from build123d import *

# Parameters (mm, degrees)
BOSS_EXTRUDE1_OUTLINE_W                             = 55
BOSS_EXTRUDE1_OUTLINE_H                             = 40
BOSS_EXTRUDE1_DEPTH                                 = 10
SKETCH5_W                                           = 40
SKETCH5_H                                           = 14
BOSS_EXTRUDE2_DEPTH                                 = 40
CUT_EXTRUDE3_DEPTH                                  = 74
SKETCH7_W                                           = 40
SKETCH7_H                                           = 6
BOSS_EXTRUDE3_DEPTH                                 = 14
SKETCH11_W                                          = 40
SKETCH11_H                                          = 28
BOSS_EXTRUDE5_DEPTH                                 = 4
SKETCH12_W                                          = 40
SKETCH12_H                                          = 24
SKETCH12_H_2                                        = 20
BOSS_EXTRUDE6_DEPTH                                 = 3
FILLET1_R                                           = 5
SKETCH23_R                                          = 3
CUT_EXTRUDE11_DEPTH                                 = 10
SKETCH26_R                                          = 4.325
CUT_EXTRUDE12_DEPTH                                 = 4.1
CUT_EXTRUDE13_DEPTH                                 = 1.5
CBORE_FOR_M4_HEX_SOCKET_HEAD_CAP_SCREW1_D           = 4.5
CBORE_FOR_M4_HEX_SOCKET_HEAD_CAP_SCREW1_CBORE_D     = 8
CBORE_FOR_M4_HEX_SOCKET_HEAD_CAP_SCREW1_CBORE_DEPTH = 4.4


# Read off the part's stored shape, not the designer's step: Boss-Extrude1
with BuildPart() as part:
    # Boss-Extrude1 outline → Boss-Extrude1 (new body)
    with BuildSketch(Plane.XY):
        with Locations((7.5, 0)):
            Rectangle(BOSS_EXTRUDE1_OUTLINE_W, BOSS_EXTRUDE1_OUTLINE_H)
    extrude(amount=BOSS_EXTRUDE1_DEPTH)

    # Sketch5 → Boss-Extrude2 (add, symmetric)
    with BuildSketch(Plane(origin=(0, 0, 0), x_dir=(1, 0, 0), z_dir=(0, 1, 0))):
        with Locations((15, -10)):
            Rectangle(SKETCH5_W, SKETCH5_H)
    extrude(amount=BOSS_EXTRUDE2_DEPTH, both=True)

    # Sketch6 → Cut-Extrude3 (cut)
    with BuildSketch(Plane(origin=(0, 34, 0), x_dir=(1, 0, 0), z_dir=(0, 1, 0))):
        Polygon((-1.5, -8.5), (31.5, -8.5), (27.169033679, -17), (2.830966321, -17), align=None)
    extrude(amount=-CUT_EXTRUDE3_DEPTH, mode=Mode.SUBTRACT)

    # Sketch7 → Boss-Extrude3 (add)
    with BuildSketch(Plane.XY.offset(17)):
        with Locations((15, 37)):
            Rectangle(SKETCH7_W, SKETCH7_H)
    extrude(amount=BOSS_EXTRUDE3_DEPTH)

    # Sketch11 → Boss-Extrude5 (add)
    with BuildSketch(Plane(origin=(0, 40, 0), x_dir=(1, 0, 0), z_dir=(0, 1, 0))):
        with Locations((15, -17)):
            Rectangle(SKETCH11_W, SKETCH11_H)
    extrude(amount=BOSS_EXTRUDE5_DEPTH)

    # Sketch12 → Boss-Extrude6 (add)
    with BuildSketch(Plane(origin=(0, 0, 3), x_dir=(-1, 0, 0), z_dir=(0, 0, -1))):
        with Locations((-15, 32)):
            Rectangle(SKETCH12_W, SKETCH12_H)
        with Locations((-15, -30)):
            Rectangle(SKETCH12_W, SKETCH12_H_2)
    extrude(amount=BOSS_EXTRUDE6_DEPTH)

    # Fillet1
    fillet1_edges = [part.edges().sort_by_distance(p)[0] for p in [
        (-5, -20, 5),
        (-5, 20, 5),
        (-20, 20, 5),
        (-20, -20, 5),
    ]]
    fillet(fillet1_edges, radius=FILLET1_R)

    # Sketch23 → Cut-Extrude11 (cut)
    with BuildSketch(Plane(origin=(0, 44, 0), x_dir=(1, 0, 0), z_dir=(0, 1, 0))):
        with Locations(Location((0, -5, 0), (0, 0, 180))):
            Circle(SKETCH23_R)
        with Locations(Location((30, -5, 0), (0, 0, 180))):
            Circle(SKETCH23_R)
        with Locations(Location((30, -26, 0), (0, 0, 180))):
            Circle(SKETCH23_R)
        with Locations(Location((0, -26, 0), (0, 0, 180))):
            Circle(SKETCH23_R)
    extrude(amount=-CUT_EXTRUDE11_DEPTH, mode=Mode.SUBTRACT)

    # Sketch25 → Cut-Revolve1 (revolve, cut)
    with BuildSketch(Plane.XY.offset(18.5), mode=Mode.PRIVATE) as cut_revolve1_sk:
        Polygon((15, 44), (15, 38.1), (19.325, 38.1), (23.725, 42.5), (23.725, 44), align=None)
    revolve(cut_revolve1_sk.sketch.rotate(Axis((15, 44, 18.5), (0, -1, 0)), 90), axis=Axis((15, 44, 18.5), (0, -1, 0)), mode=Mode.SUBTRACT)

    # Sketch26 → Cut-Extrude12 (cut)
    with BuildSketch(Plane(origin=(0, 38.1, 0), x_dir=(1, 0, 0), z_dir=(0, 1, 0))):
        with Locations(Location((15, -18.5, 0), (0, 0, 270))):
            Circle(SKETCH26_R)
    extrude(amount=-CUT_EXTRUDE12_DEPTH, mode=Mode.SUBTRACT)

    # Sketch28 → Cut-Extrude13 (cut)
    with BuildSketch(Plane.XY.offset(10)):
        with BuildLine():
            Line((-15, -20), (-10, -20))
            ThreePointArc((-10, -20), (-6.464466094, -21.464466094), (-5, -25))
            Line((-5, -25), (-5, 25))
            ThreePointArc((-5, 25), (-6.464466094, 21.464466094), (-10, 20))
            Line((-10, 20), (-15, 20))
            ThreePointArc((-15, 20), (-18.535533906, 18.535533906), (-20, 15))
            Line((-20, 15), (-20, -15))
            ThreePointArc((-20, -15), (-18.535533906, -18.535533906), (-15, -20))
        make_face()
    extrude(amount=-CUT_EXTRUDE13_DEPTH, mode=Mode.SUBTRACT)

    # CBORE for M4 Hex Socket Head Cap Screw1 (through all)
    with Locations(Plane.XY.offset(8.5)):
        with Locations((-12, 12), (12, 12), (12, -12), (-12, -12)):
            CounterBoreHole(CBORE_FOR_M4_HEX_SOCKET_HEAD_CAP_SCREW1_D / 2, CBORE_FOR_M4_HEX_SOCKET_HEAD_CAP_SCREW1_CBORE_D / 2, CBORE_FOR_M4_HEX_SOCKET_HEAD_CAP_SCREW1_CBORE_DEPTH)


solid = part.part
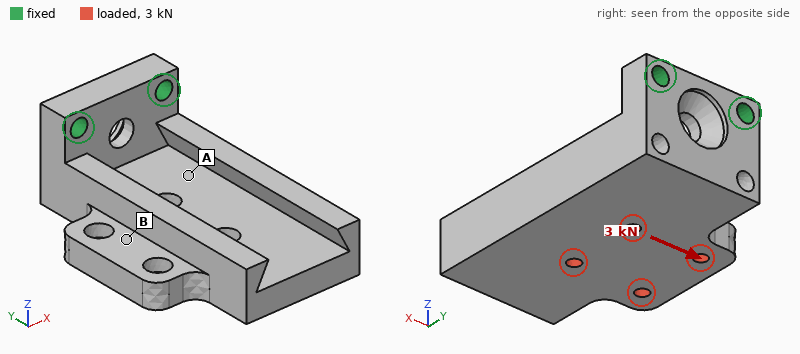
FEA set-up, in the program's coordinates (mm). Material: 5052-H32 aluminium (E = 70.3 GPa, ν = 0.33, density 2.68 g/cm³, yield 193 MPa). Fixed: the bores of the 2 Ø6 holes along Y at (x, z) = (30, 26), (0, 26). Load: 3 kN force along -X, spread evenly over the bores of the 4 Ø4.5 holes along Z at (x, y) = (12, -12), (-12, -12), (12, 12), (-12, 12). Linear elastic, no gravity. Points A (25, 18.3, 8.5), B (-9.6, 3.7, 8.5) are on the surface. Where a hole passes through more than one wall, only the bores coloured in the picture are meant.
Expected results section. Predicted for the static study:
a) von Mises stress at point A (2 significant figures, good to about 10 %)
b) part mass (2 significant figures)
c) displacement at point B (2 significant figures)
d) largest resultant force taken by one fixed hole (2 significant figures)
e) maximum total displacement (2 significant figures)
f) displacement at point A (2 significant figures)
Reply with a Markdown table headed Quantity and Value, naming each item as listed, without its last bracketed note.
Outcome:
| Quantity | Value |
|---|---|
| von Mises stress at point A | 35 MPa |
| part mass | 120 g |
| displacement at point B | 0.14 mm |
| largest resultant force taken by one fixed hole | 4.3 kN |
| maximum total displacement | 0.28 mm |
| displacement at point A | 0.079 mm |
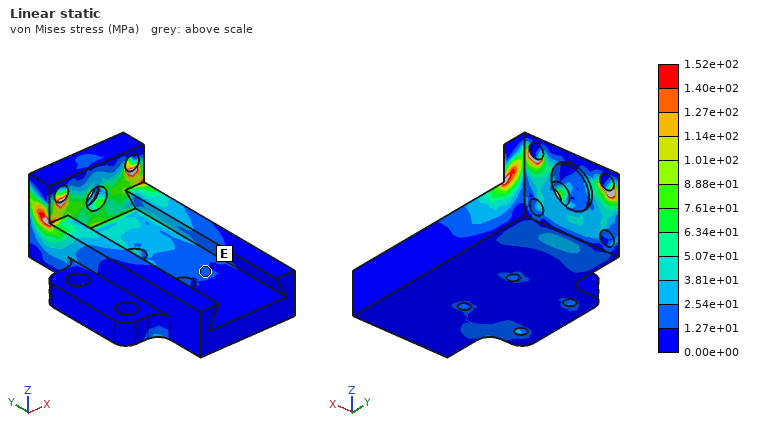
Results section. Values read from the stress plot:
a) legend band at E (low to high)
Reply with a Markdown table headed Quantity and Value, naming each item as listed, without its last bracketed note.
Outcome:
| Quantity | Value |
|---|---|
| legend band at E | 1.27e+01 to 2.54e+01 MPa |
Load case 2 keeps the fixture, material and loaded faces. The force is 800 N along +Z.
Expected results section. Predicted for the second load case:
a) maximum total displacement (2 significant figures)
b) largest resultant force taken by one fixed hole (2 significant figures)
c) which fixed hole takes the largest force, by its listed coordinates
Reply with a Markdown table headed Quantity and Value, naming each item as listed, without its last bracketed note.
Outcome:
| Quantity | Value |
|---|---|
| maximum total displacement | 0.31 mm |
| largest resultant force taken by one fixed hole | 780 N |
| which fixed hole takes the largest force, by its listed coordinates | (0, 26) |
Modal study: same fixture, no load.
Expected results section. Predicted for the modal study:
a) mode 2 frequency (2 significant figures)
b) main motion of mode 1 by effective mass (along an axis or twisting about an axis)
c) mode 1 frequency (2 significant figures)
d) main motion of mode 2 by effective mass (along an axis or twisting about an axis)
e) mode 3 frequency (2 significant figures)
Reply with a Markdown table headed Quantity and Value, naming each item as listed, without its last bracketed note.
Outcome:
| Quantity | Value |
|---|---|
| mode 2 frequency | 1800 Hz |
| main motion of mode 1 by effective mass | along Z |
| mode 1 frequency | 1000 Hz |
| main motion of mode 2 by effective mass | along X |
| mode 3 frequency | 3900 Hz |
